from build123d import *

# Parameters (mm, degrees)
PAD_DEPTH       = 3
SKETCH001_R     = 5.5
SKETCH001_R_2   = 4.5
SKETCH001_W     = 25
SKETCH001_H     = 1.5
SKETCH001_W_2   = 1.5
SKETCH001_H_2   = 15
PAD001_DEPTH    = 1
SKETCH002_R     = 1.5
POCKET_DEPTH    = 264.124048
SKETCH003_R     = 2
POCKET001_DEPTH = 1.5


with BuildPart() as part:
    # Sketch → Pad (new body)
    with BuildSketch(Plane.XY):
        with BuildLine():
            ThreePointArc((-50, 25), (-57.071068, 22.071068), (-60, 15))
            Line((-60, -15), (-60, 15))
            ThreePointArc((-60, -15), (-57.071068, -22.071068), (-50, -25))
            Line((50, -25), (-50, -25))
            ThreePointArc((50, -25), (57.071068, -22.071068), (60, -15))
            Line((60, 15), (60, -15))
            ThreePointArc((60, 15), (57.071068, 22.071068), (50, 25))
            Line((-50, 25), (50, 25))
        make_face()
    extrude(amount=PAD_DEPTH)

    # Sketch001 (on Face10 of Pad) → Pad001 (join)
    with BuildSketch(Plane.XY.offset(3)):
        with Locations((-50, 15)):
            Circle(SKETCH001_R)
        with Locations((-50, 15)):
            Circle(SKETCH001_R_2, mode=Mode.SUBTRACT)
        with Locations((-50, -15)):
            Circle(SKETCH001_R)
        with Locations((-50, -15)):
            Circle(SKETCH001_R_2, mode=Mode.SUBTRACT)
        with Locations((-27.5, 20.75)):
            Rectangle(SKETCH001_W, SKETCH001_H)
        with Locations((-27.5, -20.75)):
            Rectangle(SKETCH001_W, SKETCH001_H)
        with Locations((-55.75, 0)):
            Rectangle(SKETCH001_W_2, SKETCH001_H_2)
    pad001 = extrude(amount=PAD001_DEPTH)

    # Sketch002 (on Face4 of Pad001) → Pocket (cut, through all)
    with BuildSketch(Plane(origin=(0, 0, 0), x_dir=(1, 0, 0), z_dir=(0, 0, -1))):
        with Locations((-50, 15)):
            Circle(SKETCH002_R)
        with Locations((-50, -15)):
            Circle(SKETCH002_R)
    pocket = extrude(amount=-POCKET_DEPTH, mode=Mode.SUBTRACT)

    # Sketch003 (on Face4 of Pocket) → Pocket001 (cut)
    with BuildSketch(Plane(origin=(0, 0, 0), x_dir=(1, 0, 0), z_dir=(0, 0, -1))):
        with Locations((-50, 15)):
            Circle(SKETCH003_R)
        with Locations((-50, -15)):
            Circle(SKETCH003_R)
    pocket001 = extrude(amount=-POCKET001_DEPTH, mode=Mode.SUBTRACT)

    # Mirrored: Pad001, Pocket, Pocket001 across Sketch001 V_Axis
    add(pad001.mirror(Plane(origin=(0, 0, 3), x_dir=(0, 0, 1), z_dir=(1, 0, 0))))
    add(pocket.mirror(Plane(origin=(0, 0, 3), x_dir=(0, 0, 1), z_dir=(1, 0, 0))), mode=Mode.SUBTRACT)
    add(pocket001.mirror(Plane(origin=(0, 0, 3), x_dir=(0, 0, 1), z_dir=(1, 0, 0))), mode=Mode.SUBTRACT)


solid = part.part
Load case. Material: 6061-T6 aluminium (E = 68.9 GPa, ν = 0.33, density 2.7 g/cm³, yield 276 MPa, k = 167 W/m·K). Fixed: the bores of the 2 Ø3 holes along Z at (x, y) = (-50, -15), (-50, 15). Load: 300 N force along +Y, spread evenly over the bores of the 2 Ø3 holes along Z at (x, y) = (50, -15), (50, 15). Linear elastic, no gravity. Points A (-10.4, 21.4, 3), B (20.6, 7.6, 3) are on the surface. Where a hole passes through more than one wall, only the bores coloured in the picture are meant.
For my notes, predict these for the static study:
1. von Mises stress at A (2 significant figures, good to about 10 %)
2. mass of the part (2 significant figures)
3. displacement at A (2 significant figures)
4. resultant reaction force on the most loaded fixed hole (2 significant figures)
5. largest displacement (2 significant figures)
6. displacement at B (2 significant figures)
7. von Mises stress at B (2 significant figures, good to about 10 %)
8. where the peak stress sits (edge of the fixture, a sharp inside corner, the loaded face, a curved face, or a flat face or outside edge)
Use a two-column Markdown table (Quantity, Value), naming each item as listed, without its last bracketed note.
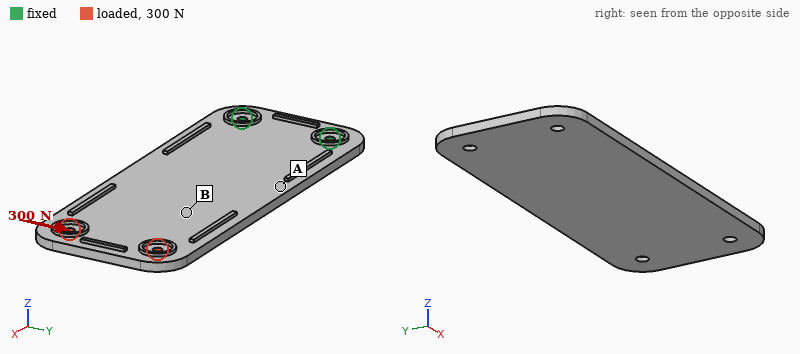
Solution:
| Quantity | Value |
|---|---|
| von Mises stress at A | 14 MPa |
| mass of the part | 48 g |
| displacement at A | 0.039 mm |
| resultant reaction force on the most loaded fixed hole | 980 N |
| largest displacement | 0.11 mm |
| displacement at B | 0.053 mm |
| von Mises stress at B | 7.5 MPa |
| where the peak stress sits | edge of the fixture |
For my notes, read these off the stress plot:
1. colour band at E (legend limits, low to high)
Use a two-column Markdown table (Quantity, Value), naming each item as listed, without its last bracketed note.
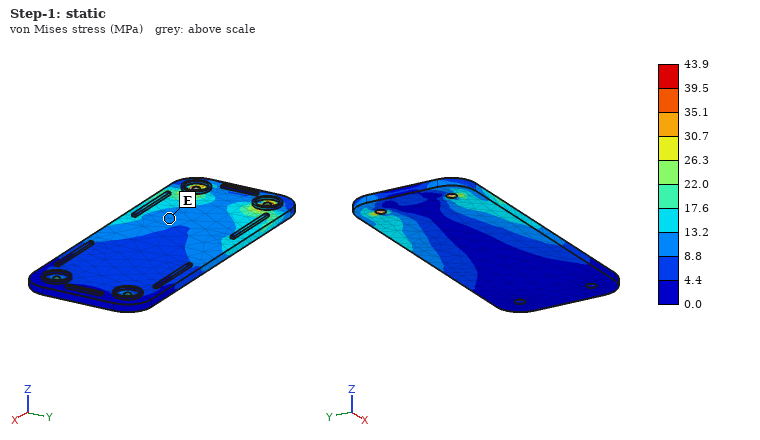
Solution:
| Quantity | Value |
|---|---|
| colour band at E | 8.8 to 13.2 MPa |
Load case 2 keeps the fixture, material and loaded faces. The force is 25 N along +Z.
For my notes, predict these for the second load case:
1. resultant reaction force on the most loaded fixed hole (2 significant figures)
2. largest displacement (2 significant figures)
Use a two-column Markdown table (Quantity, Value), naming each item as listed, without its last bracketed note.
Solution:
| Quantity | Value |
|---|---|
| resultant reaction force on the most loaded fixed hole | 40 N |
| largest displacement | 1.4 mm |
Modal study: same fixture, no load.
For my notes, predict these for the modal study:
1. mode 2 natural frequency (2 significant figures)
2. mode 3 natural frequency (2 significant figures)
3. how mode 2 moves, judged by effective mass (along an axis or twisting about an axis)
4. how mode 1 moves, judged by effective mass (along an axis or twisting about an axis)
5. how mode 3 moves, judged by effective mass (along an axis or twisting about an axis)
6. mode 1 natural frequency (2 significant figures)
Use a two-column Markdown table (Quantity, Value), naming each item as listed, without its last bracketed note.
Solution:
| Quantity | Value |
|---|---|
| mode 2 natural frequency | 920 Hz |
| mode 3 natural frequency | 1200 Hz |
| how mode 2 moves, judged by effective mass | twisting about X |
| how mode 1 moves, judged by effective mass | along Z |
| how mode 3 moves, judged by effective mass | along Z |
| mode 1 natural frequency | 190 Hz |
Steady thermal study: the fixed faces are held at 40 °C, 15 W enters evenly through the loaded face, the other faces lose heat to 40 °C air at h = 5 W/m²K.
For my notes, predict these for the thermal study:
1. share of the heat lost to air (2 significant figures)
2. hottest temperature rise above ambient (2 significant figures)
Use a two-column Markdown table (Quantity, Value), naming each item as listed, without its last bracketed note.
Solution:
| Quantity | Value |
|---|---|
| share of the heat lost to air | 13 % |
| hottest temperature rise above ambient | 62 K |
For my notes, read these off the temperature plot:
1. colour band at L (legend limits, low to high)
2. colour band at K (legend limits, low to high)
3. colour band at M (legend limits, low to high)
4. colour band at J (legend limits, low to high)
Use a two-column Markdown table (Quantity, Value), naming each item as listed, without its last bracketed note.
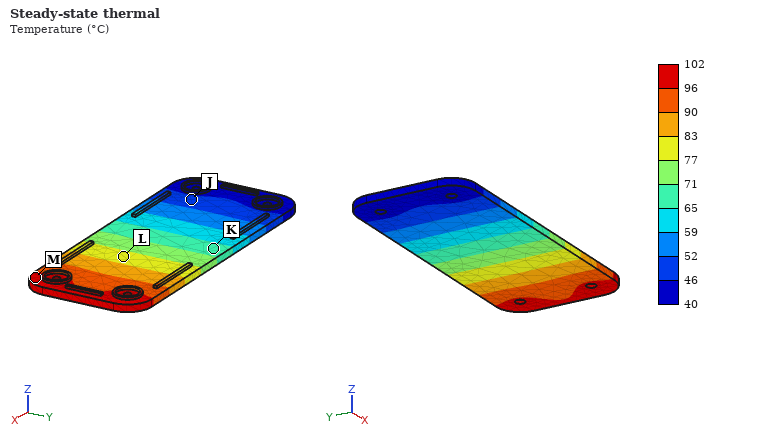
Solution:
| Quantity | Value |
|---|---|
| colour band at L | 77 to 83 °C |
| colour band at K | 65 to 71 °C |
| colour band at M | 96 to 102 °C |
| colour band at J | 46 to 52 °C |
